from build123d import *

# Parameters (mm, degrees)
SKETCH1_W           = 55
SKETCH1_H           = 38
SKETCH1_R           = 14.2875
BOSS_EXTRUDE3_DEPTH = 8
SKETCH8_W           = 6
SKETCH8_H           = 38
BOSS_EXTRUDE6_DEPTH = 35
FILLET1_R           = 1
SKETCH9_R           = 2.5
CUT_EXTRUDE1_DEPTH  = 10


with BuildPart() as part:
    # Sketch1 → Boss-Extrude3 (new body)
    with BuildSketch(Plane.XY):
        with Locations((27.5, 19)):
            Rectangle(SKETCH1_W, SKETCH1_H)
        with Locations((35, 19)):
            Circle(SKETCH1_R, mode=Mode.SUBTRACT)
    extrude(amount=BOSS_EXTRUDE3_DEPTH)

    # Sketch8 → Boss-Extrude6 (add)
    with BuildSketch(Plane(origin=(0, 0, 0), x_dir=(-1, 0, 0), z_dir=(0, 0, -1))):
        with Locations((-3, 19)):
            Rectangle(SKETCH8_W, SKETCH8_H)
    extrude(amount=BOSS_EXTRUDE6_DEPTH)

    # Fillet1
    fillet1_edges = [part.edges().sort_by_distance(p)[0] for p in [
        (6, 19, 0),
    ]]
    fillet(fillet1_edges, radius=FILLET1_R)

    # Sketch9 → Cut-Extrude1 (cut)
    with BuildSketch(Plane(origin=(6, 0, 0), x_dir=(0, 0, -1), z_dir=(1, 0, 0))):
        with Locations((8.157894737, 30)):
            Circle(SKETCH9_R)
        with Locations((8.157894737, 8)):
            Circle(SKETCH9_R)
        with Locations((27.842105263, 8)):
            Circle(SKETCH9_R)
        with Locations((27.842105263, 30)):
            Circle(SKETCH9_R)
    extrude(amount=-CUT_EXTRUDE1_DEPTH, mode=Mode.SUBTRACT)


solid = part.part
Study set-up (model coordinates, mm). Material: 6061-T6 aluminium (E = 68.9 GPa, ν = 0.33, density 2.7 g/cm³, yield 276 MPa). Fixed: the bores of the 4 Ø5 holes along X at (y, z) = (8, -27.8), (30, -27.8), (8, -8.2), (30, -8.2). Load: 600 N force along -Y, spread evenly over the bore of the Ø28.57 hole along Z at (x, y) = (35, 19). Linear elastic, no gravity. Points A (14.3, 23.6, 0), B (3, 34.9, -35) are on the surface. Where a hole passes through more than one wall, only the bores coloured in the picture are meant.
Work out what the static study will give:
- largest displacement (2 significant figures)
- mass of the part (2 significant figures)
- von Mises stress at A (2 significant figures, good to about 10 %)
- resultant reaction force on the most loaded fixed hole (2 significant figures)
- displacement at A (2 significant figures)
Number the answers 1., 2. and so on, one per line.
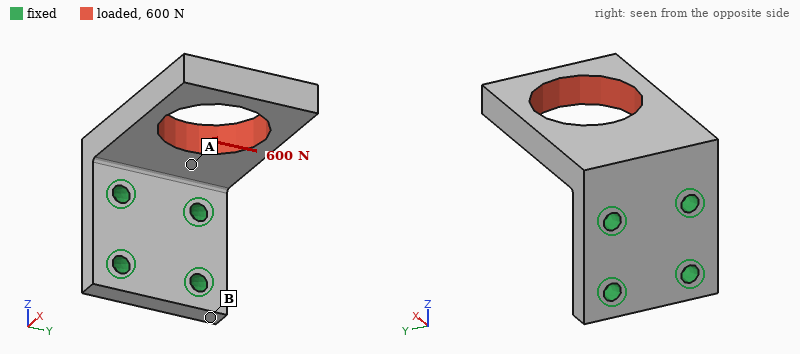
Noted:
1. 73 µm
2. 52 g
3. 16 MPa
4. 840 N
5. 12 µm
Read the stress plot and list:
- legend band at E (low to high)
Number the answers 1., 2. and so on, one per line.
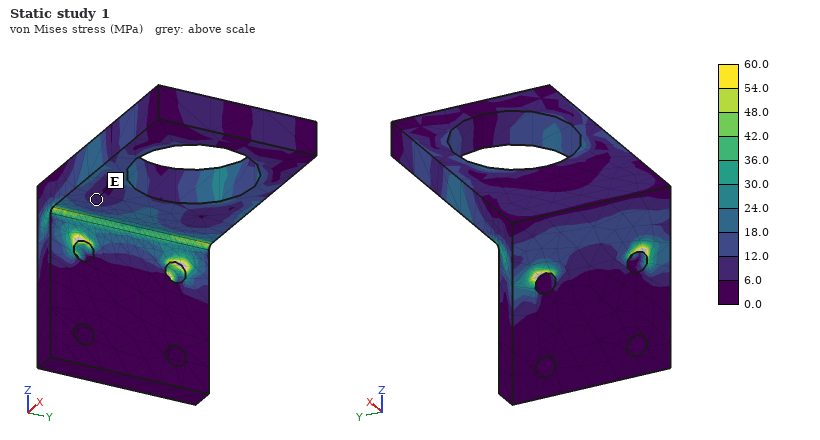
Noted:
1. 6.0 to 12.0 MPa
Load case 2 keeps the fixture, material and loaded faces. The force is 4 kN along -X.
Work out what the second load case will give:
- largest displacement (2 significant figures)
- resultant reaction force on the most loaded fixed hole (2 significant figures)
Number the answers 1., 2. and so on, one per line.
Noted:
1. 0.32 mm
2. 2.2 kN
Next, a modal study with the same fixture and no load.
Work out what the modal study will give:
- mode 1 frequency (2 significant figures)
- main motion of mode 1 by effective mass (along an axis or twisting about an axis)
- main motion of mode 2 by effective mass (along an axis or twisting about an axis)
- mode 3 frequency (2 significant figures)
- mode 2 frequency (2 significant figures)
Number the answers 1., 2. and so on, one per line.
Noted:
1. 1700 Hz
2. along Z
3. along Y
4. 5100 Hz
5. 3700 Hz
